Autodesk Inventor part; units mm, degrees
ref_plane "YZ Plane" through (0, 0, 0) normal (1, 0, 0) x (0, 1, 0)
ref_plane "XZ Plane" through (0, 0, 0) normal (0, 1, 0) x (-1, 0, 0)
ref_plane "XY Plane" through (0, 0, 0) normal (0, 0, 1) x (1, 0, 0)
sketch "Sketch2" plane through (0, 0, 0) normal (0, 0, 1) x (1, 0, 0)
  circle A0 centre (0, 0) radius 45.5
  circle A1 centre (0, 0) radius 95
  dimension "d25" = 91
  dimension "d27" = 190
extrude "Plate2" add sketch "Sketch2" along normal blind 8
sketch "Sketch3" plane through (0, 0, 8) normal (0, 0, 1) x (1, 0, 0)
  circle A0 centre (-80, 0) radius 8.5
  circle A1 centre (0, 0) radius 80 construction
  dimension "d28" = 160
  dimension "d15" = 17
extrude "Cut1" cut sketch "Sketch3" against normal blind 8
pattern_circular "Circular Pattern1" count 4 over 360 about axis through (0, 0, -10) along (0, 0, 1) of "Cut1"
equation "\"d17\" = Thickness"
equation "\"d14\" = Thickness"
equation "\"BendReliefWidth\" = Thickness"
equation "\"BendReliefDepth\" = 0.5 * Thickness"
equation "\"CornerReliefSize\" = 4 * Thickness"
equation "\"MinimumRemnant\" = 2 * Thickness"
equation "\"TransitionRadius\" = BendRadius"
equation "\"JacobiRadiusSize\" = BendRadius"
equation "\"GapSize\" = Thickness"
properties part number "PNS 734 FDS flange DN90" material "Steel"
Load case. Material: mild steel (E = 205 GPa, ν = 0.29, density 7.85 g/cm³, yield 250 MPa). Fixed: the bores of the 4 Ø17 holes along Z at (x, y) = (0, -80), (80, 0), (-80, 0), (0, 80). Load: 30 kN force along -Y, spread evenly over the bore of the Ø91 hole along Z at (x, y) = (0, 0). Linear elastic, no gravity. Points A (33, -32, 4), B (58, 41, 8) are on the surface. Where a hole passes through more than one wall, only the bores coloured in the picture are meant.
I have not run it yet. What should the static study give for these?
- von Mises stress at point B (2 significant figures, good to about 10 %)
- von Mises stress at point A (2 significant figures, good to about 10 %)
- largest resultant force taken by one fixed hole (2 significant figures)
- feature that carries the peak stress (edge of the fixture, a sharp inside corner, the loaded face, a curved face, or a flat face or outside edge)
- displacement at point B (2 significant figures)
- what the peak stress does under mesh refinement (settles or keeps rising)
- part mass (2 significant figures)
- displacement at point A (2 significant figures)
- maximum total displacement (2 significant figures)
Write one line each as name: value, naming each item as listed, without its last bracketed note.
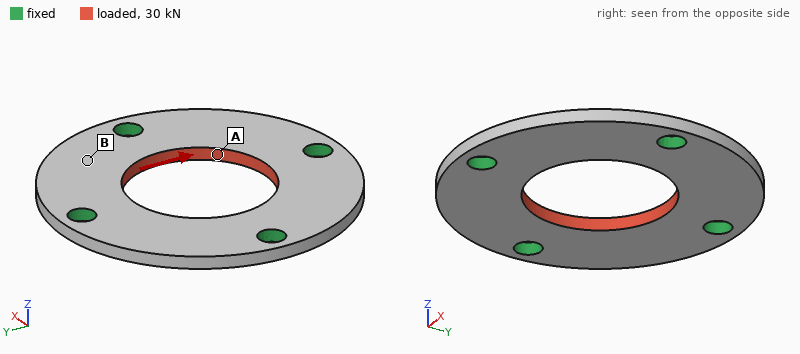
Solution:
von Mises stress at point B: 8.9 MPa
von Mises stress at point A: 20 MPa
largest resultant force taken by one fixed hole: 7.7 kN
feature that carries the peak stress: edge of the fixture
displacement at point B: 4.6 µm
what the peak stress does under mesh refinement: keeps rising
part mass: 1.3 kg
displacement at point A: 6.3 µm
maximum total displacement: 6.5 µm
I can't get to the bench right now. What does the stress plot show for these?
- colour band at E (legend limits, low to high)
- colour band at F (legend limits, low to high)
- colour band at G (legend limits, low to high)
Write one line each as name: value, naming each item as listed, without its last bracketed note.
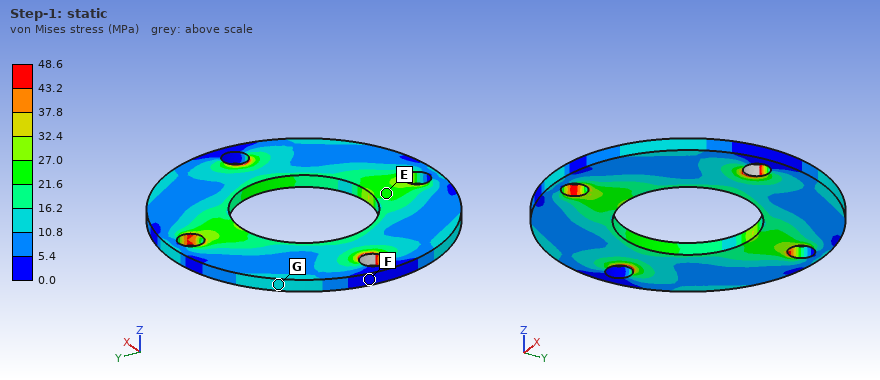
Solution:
colour band at E: 21.6 to 27.0 MPa
colour band at F: 0.0 to 5.4 MPa
colour band at G: 10.8 to 16.2 MPa
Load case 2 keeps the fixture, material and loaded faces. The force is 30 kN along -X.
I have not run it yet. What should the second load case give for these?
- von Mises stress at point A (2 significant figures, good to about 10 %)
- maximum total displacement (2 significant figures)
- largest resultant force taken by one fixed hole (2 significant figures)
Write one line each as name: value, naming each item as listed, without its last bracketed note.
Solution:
von Mises stress at point A: 20 MPa
maximum total displacement: 6.5 µm
largest resultant force taken by one fixed hole: 7.7 kN
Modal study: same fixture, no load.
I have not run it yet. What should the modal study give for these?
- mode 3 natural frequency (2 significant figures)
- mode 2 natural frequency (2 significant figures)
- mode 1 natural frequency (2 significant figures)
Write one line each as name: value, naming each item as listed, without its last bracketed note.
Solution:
mode 3 natural frequency: 3100 Hz
mode 2 natural frequency: 3100 Hz
mode 1 natural frequency: 3000 Hz
